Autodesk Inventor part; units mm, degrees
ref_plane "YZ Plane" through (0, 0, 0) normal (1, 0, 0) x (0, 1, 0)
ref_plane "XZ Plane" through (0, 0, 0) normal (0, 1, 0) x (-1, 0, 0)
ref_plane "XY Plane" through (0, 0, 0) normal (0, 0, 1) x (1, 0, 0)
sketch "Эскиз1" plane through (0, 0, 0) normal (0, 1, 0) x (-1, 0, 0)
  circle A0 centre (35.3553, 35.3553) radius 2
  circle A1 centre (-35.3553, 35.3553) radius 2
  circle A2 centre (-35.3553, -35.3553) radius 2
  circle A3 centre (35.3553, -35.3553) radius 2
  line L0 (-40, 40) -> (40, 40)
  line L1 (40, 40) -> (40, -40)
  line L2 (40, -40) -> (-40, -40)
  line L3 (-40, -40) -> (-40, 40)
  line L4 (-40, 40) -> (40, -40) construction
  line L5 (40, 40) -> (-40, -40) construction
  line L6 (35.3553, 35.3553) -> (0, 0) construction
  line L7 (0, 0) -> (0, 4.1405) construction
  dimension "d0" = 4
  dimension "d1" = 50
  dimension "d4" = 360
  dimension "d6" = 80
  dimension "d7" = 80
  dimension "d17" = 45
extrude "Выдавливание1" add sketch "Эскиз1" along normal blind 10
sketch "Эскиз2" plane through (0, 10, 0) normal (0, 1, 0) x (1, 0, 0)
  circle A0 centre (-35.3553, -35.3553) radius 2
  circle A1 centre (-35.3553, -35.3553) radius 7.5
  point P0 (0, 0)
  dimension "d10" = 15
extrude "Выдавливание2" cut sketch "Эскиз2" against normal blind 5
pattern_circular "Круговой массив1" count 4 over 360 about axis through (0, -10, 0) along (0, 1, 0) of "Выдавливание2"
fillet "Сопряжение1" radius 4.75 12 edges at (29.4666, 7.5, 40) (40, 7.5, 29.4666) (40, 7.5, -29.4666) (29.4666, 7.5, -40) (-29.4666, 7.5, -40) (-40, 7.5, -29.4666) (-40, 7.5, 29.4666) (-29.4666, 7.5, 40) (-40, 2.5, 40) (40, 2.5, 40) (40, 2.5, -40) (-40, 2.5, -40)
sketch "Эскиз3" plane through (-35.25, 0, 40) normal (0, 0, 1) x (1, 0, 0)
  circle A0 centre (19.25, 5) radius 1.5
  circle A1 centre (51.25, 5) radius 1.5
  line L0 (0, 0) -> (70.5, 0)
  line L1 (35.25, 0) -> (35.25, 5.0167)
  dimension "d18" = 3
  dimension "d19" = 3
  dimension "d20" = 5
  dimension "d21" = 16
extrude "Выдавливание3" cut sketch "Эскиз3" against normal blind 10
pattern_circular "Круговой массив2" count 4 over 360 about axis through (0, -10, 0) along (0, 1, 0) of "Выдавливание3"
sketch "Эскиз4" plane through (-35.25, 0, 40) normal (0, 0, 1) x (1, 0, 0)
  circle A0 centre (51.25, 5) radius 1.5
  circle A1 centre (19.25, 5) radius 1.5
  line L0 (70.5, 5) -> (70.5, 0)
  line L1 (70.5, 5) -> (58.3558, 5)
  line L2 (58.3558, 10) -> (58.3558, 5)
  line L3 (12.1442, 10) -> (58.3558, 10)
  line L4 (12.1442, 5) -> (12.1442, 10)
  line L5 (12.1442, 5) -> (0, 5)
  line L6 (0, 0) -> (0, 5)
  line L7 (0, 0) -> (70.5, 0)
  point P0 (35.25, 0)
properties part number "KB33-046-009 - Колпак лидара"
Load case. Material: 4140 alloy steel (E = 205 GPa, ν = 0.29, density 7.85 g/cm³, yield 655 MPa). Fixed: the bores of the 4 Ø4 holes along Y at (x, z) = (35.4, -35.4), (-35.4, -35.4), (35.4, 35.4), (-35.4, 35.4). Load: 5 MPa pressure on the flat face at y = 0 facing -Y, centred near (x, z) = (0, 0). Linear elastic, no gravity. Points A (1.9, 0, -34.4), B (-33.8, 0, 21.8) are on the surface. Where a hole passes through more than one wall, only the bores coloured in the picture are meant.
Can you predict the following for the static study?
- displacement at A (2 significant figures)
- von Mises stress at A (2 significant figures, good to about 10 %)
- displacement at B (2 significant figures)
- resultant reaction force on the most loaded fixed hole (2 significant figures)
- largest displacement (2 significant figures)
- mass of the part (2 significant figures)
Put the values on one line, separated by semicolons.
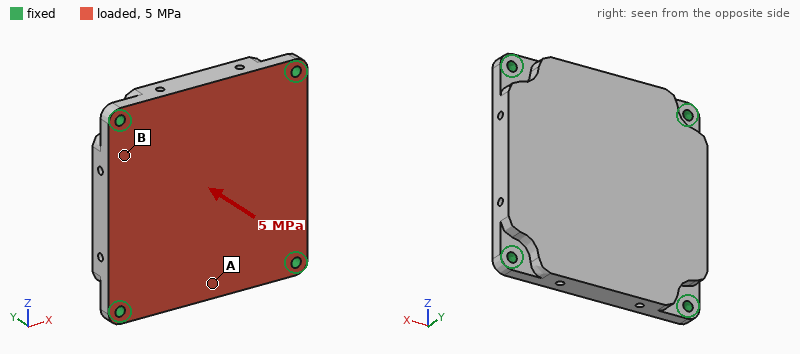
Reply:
0.070 mm; 110 MPa; 0.043 mm; 11 kN; 0.10 mm; 470 g
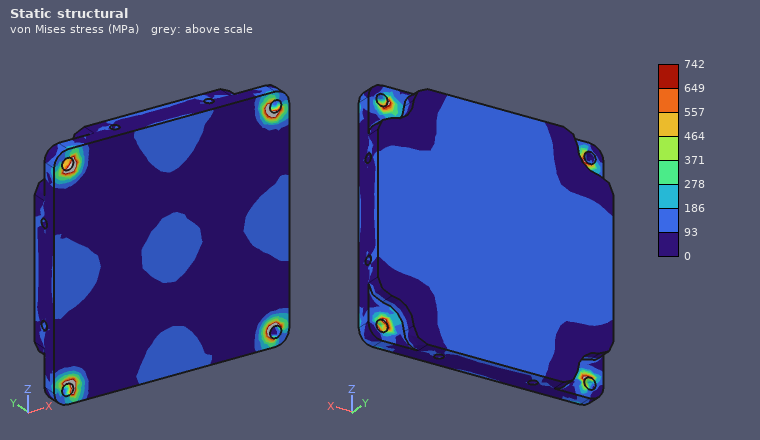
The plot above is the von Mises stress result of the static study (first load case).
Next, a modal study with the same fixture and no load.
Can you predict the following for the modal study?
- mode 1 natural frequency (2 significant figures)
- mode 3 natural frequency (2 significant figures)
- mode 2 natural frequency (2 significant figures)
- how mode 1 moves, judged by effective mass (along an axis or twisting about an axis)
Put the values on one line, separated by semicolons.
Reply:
4600 Hz; 7900 Hz; 7900 Hz; along Y
